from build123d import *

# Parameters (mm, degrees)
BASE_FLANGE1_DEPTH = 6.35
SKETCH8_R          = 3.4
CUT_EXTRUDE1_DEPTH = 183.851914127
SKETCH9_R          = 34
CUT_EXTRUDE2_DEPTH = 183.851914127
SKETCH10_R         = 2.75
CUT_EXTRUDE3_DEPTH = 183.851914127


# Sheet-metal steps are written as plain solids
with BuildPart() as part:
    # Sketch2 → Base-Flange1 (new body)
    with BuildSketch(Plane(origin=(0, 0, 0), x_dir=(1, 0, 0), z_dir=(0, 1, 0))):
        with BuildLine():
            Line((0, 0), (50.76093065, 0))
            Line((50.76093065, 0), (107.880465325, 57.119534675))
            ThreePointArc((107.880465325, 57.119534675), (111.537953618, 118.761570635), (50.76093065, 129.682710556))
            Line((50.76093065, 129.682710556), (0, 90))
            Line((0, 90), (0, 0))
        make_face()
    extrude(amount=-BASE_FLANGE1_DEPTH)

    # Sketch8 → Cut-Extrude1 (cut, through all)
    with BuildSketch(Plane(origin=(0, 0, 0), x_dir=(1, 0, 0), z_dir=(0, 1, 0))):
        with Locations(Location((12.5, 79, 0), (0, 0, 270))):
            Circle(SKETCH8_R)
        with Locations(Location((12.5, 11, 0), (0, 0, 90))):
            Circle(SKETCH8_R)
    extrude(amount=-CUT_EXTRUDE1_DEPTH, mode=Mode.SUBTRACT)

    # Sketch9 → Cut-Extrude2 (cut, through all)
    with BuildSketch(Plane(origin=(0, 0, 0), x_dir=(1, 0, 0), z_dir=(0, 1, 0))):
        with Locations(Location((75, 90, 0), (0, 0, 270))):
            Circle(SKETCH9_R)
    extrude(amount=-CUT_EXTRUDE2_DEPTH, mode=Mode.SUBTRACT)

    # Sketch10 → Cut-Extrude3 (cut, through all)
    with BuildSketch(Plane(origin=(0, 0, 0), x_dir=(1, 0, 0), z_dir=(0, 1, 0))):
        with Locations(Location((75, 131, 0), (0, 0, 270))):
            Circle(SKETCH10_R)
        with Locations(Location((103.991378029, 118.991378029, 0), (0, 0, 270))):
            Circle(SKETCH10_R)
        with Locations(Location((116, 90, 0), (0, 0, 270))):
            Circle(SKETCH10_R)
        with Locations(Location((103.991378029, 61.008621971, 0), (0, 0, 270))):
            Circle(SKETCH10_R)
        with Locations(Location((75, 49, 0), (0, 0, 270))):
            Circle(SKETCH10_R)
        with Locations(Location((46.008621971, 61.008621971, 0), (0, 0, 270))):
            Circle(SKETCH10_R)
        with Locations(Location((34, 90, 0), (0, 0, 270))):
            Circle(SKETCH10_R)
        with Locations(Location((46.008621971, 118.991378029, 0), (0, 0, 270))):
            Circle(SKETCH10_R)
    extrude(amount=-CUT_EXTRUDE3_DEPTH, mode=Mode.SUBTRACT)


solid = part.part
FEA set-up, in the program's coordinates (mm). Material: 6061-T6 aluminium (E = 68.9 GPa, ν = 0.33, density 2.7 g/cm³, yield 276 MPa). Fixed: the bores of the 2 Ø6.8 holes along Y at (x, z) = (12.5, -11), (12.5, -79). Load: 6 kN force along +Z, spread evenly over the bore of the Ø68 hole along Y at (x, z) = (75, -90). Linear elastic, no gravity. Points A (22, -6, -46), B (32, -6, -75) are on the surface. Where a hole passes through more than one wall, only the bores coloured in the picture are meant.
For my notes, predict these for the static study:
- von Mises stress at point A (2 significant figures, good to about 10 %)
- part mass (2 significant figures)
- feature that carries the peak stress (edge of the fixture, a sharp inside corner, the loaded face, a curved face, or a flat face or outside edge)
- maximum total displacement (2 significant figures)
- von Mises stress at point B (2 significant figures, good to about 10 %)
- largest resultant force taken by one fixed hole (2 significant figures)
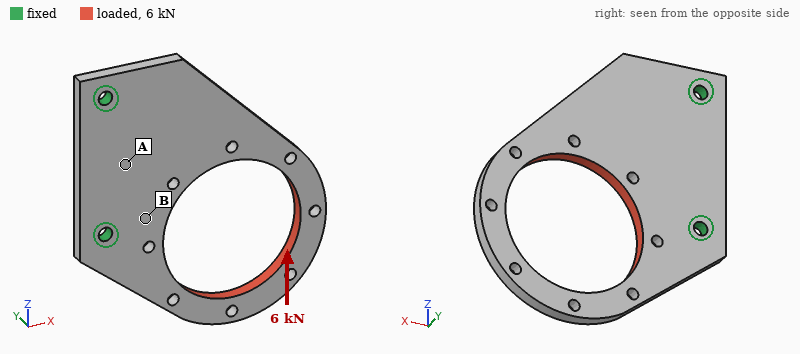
16 MPa
140 g
a curved face
0.33 mm
44 MPa
6.1 kN
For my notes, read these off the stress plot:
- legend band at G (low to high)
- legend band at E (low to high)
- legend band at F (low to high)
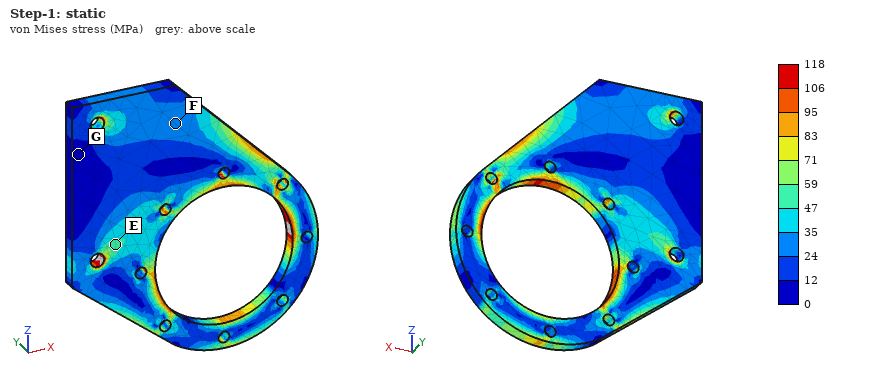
0 to 12 MPa
47 to 59 MPa
24 to 35 MPa
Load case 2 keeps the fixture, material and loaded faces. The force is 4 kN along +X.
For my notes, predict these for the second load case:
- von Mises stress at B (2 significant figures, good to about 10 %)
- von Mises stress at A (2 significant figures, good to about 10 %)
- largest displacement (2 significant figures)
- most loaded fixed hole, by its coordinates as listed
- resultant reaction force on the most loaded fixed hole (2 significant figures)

23 MPa
7.7 MPa
0.18 mm
(12.5, -79)
4.5 kN
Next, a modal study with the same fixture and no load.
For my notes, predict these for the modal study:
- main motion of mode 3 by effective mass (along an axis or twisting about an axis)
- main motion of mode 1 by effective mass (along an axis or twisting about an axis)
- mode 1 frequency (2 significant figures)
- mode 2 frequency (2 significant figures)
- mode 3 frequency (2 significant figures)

along Y
along Y
500 Hz
1000 Hz
1900 Hz
